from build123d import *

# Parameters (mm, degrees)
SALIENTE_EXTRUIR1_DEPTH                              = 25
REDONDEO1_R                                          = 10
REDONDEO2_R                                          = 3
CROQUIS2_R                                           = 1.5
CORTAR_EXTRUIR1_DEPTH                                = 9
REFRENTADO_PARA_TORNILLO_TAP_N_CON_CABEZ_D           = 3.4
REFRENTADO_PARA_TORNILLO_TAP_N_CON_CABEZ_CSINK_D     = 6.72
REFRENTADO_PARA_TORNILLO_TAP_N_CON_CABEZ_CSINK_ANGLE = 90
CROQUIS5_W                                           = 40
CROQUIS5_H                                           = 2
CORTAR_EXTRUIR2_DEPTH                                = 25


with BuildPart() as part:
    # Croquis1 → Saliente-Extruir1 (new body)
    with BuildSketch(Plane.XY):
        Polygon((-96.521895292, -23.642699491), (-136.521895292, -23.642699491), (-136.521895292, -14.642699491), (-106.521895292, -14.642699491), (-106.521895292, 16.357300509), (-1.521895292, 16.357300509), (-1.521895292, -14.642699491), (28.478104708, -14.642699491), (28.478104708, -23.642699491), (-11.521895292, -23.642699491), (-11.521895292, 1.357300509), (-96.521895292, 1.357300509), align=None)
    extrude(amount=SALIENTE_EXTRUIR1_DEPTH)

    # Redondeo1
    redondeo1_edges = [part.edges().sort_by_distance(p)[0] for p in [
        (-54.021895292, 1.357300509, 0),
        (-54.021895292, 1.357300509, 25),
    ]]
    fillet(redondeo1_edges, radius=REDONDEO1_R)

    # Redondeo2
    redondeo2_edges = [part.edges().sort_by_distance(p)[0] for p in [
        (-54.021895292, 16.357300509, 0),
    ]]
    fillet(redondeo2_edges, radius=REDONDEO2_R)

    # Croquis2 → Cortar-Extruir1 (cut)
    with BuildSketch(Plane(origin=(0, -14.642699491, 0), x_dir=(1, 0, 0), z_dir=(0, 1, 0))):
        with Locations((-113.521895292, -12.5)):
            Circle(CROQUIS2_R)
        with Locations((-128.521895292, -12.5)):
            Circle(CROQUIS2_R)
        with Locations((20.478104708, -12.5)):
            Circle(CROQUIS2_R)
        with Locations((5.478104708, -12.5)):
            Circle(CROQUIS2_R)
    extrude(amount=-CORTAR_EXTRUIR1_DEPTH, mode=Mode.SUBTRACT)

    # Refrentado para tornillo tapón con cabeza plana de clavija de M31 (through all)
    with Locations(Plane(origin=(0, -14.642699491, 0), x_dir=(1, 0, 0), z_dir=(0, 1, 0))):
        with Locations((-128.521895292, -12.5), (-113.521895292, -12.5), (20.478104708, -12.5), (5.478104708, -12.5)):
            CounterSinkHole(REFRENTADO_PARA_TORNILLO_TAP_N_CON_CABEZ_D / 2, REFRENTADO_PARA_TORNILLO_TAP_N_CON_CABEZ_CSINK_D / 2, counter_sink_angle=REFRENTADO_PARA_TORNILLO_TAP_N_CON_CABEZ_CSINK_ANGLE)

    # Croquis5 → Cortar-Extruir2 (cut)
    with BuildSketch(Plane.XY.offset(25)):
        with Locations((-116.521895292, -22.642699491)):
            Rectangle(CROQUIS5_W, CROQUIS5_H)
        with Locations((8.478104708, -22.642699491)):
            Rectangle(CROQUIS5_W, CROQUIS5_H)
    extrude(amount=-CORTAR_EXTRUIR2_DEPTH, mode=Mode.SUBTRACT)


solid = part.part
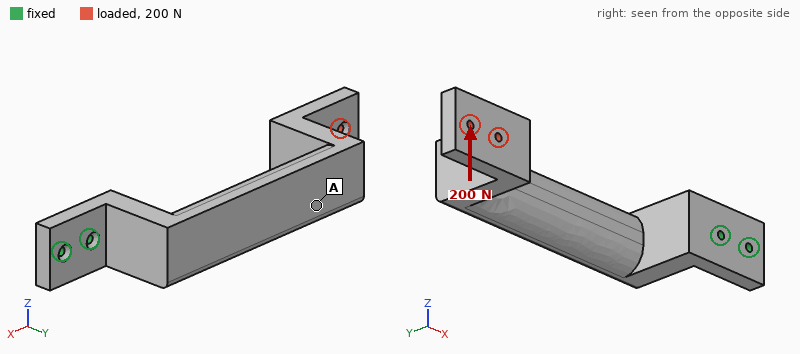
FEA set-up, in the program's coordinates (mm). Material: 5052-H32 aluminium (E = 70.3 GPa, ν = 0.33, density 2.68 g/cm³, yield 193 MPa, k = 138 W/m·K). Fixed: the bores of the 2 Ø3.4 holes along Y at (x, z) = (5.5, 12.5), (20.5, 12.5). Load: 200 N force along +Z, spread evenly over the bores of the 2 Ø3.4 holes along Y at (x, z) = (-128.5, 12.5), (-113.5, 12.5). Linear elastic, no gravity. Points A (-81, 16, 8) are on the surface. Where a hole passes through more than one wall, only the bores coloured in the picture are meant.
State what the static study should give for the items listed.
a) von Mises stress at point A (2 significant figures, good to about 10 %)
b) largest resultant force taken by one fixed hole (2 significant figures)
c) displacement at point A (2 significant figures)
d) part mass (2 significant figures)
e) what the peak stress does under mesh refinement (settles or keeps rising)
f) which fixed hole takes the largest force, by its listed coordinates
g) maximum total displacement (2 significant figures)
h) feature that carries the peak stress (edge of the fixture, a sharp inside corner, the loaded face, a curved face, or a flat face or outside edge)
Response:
6.5 MPa
1.6 kN
0.31 mm
150 g
keeps rising
(5.5, 12.5)
0.68 mm
edge of the fixture
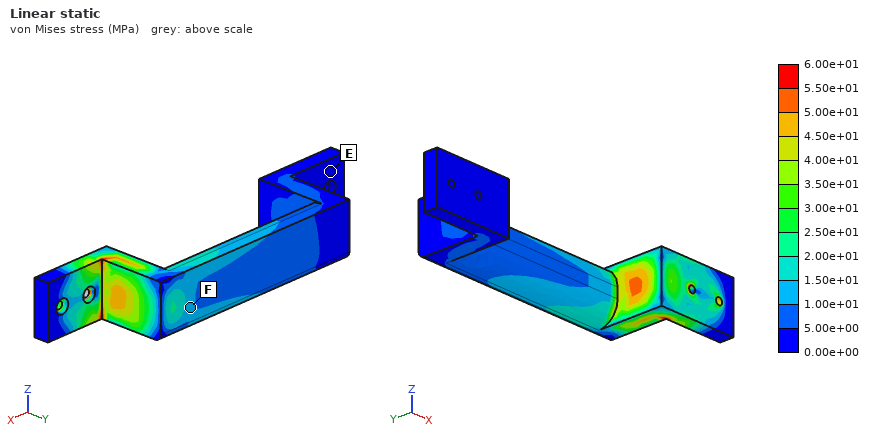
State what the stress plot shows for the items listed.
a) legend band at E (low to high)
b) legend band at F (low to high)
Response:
0.00e+00 to 5.00e+00 MPa
1.00e+01 to 1.50e+01 MPa
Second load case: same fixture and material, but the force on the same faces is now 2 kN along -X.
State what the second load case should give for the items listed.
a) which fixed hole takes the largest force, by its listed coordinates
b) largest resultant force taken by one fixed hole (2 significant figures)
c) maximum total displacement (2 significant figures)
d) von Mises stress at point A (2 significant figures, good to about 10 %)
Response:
(5.5, 12.5)
1.5 kN
2.0 mm
66 MPa
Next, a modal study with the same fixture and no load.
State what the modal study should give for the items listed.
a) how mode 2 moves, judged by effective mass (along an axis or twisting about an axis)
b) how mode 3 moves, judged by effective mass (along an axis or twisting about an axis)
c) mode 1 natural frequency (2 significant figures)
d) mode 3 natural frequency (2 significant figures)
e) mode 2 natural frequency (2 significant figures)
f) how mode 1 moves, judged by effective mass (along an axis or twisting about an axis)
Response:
along Z
along Z
270 Hz
1400 Hz
450 Hz
along Y
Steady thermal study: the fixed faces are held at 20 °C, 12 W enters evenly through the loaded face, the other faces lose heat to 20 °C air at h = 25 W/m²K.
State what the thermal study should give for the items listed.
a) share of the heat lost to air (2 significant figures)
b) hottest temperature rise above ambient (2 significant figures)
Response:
49 %
37 K
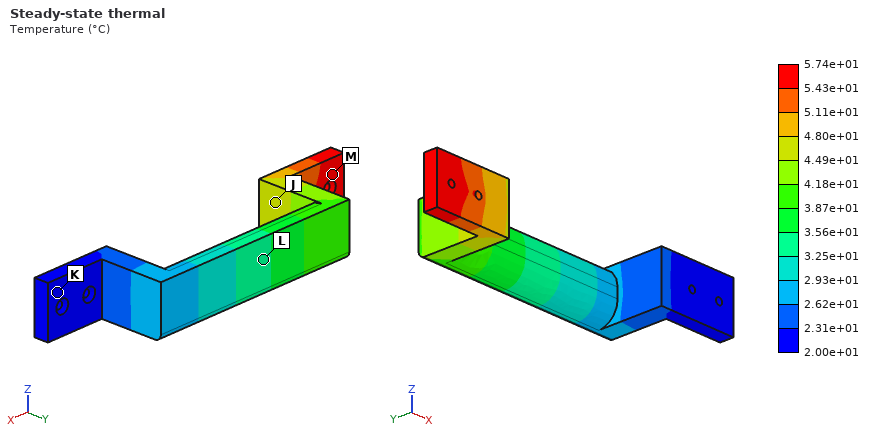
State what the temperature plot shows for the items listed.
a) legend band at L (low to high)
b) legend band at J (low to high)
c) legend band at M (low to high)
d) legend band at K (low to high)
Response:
3.25e+01 to 3.56e+01 °C
4.49e+01 to 4.80e+01 °C
5.43e+01 to 5.74e+01 °C
2.00e+01 to 2.31e+01 °C
